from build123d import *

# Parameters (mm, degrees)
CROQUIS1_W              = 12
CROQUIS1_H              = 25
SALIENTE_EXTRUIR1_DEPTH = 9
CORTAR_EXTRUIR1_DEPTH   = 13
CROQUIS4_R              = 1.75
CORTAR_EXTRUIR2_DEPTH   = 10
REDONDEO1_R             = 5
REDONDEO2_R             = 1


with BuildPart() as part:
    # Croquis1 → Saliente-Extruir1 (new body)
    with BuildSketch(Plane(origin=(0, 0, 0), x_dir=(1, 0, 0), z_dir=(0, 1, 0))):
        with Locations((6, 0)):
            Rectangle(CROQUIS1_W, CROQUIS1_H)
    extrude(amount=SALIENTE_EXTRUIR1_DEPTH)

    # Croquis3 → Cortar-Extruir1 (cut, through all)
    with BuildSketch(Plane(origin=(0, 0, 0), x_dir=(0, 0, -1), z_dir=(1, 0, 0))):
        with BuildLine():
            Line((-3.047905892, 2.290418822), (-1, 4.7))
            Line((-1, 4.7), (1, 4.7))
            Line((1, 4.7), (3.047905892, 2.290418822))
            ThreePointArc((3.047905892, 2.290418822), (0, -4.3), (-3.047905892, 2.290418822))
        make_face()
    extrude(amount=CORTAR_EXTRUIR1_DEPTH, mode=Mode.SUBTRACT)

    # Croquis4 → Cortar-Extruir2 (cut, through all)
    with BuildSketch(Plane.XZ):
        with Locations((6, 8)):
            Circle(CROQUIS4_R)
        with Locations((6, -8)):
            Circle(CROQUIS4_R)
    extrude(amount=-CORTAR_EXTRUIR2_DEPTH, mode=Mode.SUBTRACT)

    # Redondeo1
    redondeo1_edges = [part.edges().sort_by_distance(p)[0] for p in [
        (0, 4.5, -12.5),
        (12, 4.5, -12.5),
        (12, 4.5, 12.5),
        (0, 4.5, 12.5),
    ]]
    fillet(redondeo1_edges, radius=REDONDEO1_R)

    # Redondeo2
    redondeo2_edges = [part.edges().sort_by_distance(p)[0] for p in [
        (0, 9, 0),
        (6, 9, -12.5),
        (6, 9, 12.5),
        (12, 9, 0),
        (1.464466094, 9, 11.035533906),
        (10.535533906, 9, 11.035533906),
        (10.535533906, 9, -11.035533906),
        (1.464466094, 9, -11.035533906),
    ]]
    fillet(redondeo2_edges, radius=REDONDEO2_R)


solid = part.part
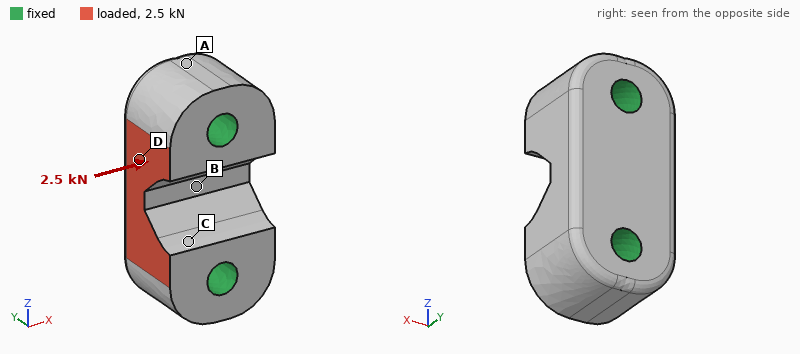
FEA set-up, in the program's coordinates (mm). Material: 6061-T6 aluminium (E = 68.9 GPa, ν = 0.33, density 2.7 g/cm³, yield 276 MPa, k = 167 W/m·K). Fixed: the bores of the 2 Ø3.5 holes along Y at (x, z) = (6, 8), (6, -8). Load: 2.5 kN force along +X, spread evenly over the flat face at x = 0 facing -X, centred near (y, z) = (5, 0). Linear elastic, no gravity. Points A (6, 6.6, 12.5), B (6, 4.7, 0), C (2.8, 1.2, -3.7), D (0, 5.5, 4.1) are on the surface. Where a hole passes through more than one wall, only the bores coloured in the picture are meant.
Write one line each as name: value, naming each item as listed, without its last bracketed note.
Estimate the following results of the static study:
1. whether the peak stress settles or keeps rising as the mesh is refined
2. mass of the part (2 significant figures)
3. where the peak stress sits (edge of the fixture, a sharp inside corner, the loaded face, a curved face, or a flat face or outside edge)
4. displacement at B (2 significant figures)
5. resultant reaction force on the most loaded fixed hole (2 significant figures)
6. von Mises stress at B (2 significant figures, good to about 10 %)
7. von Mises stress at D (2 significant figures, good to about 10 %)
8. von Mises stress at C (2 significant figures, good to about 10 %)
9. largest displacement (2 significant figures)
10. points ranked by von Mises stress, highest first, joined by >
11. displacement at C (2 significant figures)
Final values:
whether the peak stress settles or keeps rising as the mesh is refined: keeps rising
mass of the part: 5.4 g
where the peak stress sits: edge of the fixture
displacement at B: 2.5 µm
resultant reaction force on the most loaded fixed hole: 1.3 kN
von Mises stress at B: 13 MPa
von Mises stress at D: 20 MPa
von Mises stress at C: 26 MPa
largest displacement: 4.3 µm
points ranked by von Mises stress, highest first, joined by >: C > D > B > A
displacement at C: 2.6 µm
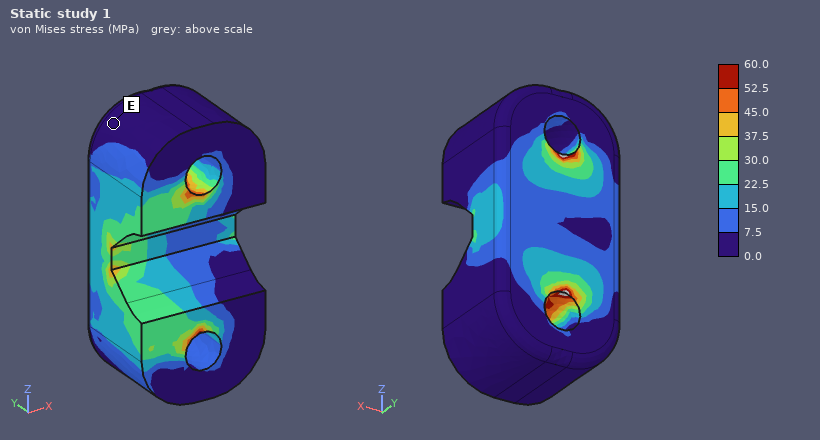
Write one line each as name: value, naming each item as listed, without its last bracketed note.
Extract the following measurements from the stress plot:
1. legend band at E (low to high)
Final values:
legend band at E: 0.0 to 7.5 MPa
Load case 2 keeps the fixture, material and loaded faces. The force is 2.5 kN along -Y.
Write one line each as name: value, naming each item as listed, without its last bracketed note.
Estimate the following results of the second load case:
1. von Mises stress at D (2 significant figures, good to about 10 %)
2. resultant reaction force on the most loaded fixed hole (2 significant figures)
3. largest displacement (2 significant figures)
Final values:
von Mises stress at D: 63 MPa
resultant reaction force on the most loaded fixed hole: 1.3 kN
largest displacement: 12 µm
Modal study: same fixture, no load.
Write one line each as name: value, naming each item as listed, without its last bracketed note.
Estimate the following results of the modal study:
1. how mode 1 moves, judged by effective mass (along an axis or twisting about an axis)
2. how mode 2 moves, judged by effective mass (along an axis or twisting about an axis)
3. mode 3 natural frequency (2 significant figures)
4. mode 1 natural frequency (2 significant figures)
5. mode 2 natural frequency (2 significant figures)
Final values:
how mode 1 moves, judged by effective mass: along X
how mode 2 moves, judged by effective mass: along Y
mode 3 natural frequency: 100 kHz
mode 1 natural frequency: 81 kHz
mode 2 natural frequency: 90 kHz
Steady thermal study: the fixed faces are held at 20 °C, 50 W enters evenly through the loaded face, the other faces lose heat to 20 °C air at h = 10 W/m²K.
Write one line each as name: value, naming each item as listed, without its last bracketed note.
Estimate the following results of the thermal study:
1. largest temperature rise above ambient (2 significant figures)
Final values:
largest temperature rise above ambient: 17 K
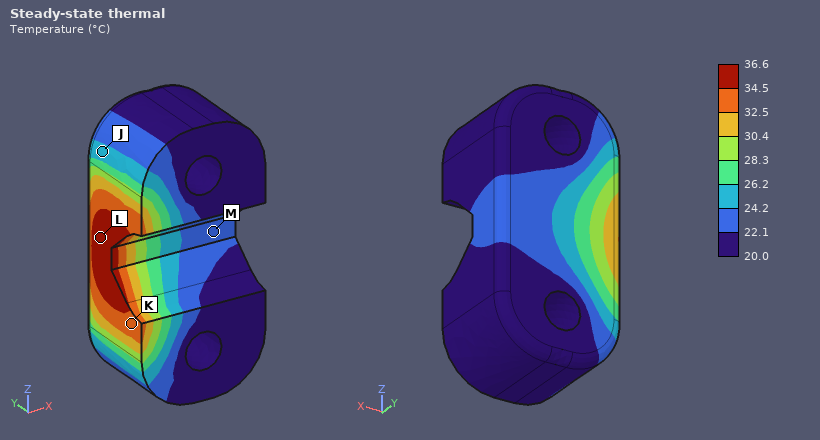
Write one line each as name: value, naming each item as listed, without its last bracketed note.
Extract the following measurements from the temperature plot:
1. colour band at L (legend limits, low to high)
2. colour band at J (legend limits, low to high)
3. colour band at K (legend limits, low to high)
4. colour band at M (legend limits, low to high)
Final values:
colour band at L: 34.5 to 36.6 °C
colour band at J: 24.2 to 26.2 °C
colour band at K: 32.5 to 34.5 °C
colour band at M: 22.1 to 24.2 °C
